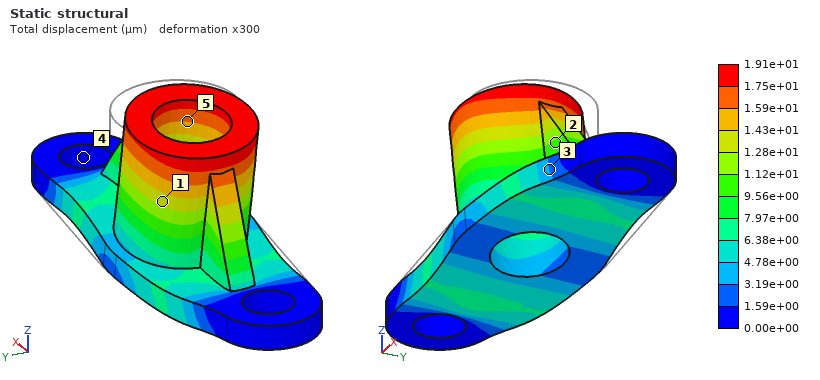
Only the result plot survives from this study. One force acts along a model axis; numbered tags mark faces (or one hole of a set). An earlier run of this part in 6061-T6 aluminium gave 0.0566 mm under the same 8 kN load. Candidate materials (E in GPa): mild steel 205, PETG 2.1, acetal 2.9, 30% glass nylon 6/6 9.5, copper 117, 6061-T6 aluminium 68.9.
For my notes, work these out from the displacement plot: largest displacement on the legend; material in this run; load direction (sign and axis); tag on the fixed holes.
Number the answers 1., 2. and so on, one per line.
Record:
1. 1.91e+01 µm
2. mild steel
3. -X
4. 4
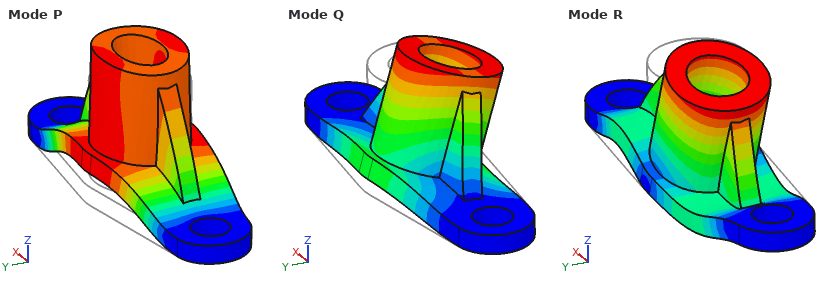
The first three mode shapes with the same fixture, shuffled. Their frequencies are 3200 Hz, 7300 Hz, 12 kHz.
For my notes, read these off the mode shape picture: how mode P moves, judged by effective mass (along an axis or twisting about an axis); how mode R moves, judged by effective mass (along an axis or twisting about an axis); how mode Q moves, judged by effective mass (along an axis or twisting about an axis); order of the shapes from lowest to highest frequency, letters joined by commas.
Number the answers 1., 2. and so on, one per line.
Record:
1. along Z
2. along X
3. along Y
4. Q, P, R
